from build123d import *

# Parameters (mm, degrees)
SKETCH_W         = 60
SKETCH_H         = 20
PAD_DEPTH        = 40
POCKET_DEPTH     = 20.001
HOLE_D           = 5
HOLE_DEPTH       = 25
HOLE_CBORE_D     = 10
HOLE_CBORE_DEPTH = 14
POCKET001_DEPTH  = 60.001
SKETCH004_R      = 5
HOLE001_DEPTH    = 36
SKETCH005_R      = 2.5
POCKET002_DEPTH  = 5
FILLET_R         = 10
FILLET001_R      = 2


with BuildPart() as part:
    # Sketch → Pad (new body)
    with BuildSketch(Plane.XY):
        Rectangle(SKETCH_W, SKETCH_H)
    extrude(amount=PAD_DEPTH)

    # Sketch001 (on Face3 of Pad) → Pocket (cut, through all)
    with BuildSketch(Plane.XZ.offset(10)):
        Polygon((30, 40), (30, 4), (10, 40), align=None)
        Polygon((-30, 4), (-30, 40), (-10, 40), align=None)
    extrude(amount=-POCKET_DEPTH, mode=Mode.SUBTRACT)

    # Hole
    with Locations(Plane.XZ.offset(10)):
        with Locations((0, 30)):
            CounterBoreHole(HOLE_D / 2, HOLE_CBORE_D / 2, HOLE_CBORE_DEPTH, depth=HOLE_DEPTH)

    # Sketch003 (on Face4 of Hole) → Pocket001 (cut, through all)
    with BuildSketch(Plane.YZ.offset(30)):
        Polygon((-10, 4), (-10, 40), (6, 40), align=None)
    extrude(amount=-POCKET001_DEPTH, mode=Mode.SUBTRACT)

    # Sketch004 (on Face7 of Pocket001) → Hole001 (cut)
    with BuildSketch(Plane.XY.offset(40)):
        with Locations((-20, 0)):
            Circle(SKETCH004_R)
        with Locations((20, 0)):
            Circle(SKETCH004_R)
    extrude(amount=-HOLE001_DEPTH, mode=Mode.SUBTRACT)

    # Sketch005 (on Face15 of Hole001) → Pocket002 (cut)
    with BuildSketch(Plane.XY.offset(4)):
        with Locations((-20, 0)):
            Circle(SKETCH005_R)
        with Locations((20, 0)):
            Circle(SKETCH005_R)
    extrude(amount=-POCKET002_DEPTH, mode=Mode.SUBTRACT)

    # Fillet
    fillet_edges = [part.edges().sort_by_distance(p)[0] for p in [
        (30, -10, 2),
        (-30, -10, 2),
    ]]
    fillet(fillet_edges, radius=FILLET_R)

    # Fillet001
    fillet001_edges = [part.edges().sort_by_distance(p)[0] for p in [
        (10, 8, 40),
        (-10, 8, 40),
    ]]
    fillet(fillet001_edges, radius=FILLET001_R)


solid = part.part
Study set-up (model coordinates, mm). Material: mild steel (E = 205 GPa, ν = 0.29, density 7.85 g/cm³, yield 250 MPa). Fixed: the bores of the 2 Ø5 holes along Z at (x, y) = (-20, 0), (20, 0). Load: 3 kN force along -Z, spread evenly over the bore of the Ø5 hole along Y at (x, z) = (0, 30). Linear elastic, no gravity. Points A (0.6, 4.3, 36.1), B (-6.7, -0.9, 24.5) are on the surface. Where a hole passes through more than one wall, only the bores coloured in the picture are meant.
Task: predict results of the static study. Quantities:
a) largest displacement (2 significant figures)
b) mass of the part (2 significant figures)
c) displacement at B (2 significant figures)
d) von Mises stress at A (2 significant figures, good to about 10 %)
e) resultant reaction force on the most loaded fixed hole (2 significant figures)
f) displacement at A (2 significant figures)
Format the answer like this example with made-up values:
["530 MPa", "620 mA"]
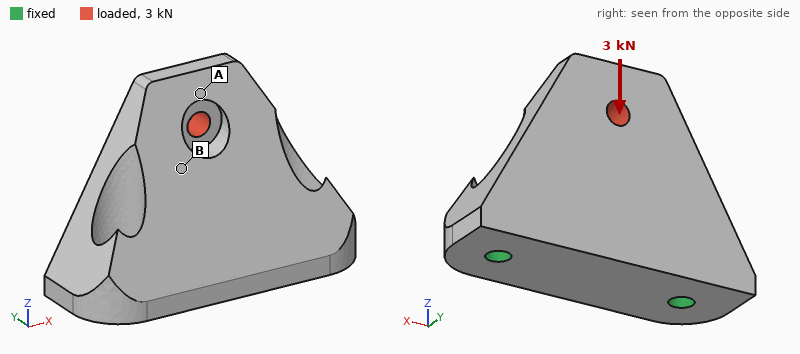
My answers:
["32 µm", "160 g", "17 µm", "34 MPa", "1.6 kN", "27 µm"]
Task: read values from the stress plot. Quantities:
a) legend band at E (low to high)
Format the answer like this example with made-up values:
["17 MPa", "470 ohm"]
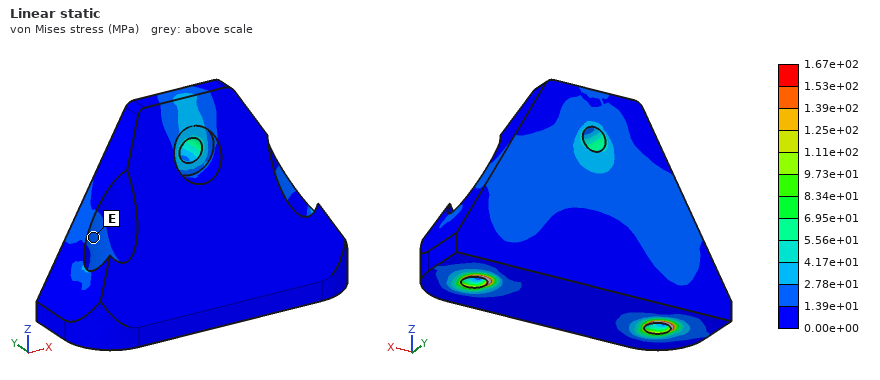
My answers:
["1.39e+01 to 2.78e+01 MPa"]
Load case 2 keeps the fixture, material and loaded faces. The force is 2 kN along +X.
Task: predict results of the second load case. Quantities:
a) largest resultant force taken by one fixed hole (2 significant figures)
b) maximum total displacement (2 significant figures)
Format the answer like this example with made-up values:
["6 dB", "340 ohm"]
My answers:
["1.7 kN", "6.1 µm"]
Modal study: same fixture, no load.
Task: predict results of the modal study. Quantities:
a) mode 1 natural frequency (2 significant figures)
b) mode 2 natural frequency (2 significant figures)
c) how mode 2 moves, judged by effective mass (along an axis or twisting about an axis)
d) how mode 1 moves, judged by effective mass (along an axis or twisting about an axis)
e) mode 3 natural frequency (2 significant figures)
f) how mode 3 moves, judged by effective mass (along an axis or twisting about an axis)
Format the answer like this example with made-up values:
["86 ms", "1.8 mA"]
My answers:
["4100 Hz", "15 kHz", "along X", "along Y", "16 kHz", "along Z"]
